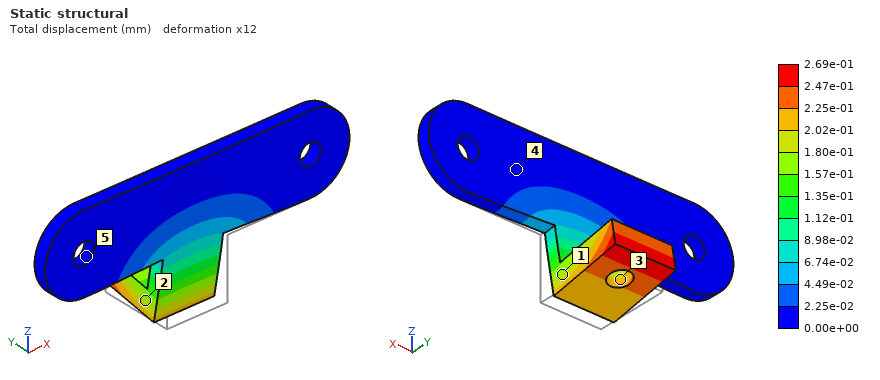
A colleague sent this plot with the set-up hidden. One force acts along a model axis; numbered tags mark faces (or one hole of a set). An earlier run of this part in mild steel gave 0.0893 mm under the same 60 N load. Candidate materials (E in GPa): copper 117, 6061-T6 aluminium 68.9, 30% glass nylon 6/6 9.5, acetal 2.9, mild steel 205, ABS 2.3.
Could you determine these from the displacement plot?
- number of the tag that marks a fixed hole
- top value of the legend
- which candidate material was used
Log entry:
5
2.69e-01 mm
6061-T6 aluminium
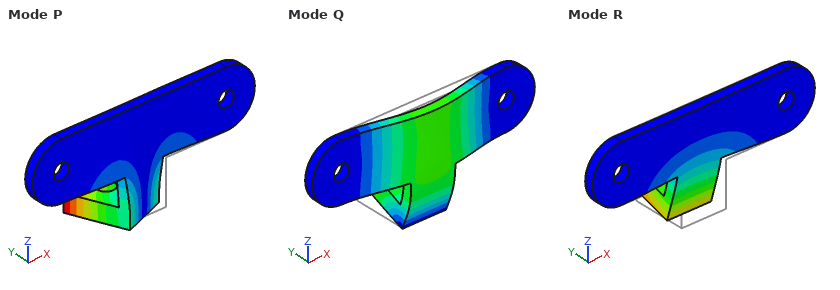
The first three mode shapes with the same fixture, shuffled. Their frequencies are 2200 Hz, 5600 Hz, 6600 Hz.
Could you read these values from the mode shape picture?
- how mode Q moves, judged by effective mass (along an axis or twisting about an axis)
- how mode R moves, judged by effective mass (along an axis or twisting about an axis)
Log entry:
along Y
along Y
